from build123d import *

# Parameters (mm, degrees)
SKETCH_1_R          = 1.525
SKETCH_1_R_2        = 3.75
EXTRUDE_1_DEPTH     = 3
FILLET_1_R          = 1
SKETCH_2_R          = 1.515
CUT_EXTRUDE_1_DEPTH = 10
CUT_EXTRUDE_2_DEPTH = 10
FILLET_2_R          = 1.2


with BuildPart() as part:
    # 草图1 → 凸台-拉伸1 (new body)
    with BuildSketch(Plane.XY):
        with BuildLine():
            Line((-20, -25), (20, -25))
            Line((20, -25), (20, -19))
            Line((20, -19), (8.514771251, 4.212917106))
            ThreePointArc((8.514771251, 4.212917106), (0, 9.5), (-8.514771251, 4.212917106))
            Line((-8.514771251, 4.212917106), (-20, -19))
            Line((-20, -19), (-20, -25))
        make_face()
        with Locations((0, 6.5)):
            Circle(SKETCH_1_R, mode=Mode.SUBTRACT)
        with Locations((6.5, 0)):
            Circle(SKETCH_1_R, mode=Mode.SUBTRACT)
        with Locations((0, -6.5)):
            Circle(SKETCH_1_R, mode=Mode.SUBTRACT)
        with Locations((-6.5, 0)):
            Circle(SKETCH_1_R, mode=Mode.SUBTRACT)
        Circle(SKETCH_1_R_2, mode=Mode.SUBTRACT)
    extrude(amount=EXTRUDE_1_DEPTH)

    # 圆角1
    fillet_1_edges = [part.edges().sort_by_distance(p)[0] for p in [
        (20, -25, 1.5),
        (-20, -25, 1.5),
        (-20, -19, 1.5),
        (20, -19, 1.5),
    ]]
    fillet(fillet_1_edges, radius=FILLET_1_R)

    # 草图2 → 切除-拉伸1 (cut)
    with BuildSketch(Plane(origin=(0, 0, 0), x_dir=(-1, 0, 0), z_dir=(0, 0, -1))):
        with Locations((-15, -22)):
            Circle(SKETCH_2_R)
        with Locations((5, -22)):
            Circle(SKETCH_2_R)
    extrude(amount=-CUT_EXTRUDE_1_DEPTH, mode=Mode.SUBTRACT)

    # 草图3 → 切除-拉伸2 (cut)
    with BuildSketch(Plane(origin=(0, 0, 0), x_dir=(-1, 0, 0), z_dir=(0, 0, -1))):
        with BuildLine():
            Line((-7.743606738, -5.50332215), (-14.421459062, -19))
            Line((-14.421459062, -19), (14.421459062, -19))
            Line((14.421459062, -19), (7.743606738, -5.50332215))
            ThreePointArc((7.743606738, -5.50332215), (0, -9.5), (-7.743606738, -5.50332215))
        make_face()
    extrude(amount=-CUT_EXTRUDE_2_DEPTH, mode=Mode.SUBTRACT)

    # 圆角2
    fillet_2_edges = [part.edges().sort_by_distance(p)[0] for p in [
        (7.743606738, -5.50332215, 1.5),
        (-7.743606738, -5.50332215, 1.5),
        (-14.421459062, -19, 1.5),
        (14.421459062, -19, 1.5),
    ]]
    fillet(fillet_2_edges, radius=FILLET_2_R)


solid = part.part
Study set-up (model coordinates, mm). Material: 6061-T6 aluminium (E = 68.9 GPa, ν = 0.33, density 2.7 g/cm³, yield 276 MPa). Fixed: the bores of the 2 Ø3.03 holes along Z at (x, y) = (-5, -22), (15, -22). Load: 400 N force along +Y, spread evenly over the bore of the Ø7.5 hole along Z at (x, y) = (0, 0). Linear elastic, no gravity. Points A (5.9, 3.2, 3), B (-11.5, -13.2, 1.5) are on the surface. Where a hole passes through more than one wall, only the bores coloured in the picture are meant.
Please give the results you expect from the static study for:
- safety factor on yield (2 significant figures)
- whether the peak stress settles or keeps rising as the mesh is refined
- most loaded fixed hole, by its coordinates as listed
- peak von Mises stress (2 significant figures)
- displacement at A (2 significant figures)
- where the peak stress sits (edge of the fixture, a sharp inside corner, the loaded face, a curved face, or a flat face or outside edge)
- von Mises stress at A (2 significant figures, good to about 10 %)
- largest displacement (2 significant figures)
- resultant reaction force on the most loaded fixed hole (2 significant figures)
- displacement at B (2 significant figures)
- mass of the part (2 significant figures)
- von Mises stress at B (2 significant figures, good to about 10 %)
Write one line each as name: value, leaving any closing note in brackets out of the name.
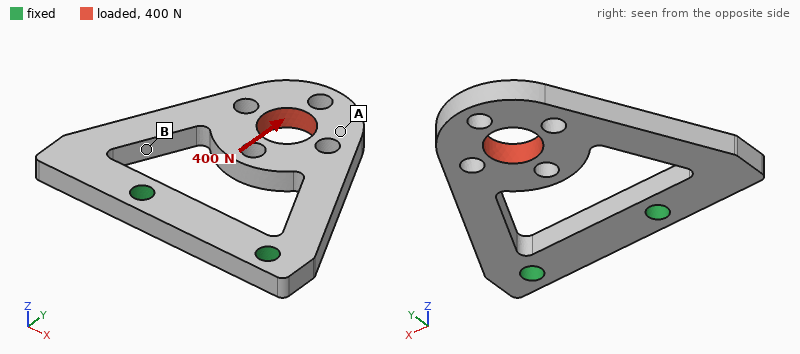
safety factor on yield: 2.4
whether the peak stress settles or keeps rising as the mesh is refined: settles
most loaded fixed hole, by its coordinates as listed: (-5, -22)
peak von Mises stress: 120 MPa
displacement at A: 29 µm
where the peak stress sits: a curved face
von Mises stress at A: 16 MPa
largest displacement: 34 µm
resultant reaction force on the most loaded fixed hole: 220 N
displacement at B: 27 µm
mass of the part: 5.1 g
von Mises stress at B: 42 MPa
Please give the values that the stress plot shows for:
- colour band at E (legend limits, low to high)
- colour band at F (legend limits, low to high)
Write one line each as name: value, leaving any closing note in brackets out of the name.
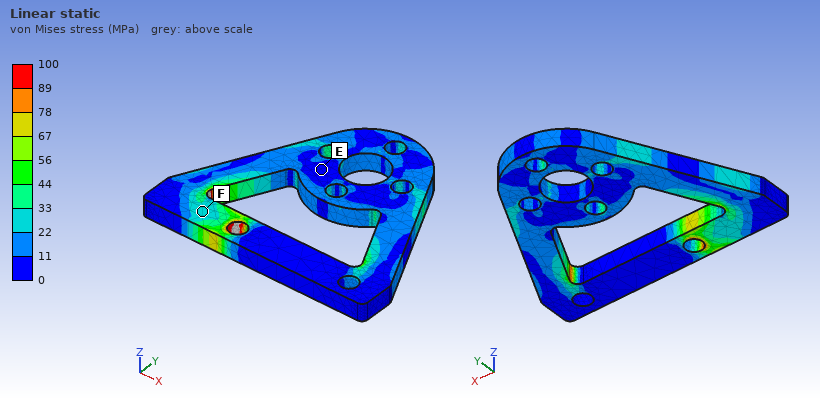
colour band at E: 0 to 11 MPa
colour band at F: 22 to 33 MPa
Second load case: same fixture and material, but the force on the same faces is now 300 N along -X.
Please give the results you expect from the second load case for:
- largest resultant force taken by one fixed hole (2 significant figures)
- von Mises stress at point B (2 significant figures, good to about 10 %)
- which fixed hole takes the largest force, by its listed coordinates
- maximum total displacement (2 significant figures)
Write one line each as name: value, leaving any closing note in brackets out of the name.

largest resultant force taken by one fixed hole: 260 N
von Mises stress at point B: 38 MPa
which fixed hole takes the largest force, by its listed coordinates: (15, -22)
maximum total displacement: 54 µm
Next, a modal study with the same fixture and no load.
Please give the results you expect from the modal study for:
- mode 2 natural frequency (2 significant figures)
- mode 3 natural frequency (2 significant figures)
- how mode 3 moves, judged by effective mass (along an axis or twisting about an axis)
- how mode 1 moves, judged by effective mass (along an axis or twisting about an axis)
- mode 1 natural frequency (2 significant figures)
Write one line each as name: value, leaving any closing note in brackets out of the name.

mode 2 natural frequency: 6400 Hz
mode 3 natural frequency: 7200 Hz
how mode 3 moves, judged by effective mass: along X
how mode 1 moves, judged by effective mass: along Z
mode 1 natural frequency: 1900 Hz
